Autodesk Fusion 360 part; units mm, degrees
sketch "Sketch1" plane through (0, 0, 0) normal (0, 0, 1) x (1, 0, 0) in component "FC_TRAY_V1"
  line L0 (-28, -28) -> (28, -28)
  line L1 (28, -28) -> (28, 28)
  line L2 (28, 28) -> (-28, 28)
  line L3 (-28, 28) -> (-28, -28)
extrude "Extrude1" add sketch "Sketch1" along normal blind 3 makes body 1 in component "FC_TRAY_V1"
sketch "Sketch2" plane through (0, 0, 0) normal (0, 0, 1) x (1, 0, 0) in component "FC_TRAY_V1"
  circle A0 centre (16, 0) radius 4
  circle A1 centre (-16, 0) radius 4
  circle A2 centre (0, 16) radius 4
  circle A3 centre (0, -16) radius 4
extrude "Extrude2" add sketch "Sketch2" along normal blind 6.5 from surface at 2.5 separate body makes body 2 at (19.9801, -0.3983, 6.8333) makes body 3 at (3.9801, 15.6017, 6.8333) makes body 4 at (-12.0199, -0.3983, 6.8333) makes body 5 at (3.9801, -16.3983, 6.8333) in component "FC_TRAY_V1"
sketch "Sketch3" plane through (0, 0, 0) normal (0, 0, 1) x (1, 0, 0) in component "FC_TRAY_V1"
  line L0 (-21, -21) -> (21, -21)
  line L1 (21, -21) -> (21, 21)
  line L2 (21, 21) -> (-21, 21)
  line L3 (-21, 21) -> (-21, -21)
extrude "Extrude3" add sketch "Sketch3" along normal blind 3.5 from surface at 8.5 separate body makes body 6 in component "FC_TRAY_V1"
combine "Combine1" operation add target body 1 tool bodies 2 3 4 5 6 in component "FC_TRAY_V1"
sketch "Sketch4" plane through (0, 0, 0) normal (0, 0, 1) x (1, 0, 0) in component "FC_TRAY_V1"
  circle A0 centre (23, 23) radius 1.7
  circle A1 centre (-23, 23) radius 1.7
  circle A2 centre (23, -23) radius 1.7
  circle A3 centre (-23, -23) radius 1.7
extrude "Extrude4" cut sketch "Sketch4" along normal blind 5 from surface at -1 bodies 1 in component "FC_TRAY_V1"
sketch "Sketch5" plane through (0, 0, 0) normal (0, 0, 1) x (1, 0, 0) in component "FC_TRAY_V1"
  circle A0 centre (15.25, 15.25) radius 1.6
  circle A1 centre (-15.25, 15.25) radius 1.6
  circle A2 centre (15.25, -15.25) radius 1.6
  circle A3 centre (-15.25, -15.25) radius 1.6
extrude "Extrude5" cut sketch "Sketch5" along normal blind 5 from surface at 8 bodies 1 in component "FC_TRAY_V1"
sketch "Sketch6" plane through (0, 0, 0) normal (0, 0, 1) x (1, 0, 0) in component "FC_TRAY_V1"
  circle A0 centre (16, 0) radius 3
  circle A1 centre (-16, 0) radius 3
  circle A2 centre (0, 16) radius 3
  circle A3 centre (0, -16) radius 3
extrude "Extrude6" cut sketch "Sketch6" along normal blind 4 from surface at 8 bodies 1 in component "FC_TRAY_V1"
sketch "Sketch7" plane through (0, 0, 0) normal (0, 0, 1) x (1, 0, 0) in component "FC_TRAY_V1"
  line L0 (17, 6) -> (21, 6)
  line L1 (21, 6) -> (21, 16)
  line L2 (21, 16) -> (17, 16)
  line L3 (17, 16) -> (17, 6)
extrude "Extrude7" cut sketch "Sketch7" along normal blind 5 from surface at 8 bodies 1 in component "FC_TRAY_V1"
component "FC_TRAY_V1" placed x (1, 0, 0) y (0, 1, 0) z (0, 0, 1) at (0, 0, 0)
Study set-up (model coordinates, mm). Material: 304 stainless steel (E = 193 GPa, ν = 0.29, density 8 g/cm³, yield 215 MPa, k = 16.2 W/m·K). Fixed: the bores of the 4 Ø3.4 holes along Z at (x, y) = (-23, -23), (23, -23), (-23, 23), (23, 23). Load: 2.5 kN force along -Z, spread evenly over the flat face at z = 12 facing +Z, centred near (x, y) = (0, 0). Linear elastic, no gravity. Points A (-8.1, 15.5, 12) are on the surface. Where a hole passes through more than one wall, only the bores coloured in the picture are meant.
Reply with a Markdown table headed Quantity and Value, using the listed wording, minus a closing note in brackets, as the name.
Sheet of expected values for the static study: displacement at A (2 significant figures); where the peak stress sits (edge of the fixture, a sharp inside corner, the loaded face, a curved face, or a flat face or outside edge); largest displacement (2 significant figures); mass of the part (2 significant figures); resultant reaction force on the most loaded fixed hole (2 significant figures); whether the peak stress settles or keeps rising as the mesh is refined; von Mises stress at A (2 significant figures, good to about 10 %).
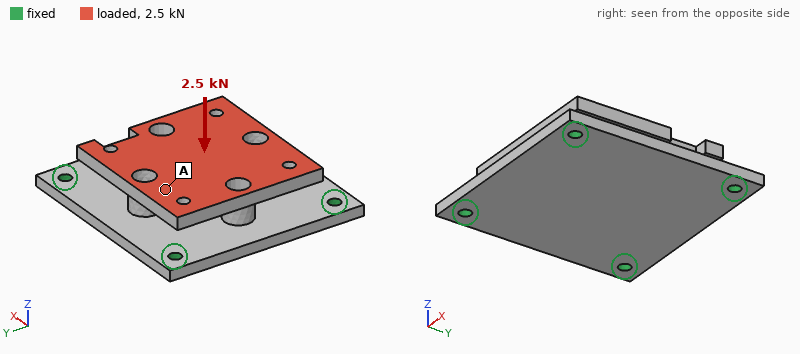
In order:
| Quantity | Value |
|---|---|
| displacement at A | 48 µm |
| where the peak stress sits | edge of the fixture |
| largest displacement | 64 µm |
| mass of the part | 130 g |
| resultant reaction force on the most loaded fixed hole | 660 N |
| whether the peak stress settles or keeps rising as the mesh is refined | keeps rising |
| von Mises stress at A | 32 MPa |
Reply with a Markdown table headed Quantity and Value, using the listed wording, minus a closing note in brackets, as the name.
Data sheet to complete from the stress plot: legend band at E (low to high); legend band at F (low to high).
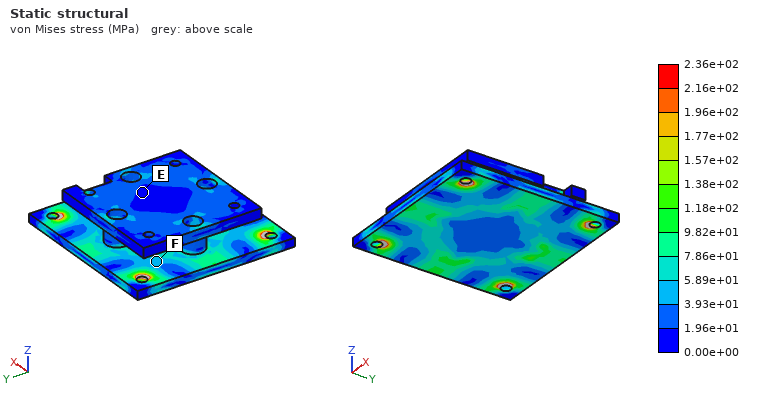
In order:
| Quantity | Value |
|---|---|
| legend band at E | 0.00e+00 to 1.96e+01 MPa |
| legend band at F | 3.93e+01 to 5.89e+01 MPa |
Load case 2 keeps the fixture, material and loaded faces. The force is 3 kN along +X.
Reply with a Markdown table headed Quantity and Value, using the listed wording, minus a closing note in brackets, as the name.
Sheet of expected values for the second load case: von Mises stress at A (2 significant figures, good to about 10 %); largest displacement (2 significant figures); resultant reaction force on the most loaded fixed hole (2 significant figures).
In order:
| Quantity | Value |
|---|---|
| von Mises stress at A | 19 MPa |
| largest displacement | 50 µm |
| resultant reaction force on the most loaded fixed hole | 900 N |
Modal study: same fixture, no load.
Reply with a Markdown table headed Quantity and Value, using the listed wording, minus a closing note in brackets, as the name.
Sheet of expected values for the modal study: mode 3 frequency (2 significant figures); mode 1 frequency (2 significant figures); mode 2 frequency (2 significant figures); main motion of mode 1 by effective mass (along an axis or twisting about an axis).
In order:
| Quantity | Value |
|---|---|
| mode 3 frequency | 5100 Hz |
| mode 1 frequency | 3800 Hz |
| mode 2 frequency | 5100 Hz |
| main motion of mode 1 by effective mass | along Z |
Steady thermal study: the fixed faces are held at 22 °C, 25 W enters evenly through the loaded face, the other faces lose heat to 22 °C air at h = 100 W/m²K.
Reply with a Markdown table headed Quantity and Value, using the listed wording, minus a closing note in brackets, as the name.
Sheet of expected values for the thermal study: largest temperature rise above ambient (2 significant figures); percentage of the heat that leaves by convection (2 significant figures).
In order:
| Quantity | Value |
|---|---|
| largest temperature rise above ambient | 64 K |
| percentage of the heat that leaves by convection | 90 % |
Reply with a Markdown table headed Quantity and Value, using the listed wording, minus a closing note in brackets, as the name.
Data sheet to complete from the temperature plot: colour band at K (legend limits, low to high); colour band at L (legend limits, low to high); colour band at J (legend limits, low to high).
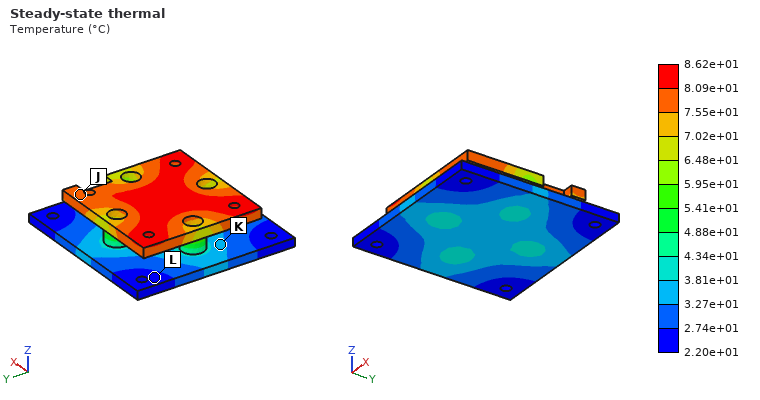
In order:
| Quantity | Value |
|---|---|
| colour band at K | 3.27e+01 to 3.81e+01 °C |
| colour band at L | 2.20e+01 to 2.74e+01 °C |
| colour band at J | 7.55e+01 to 8.09e+01 °C |
